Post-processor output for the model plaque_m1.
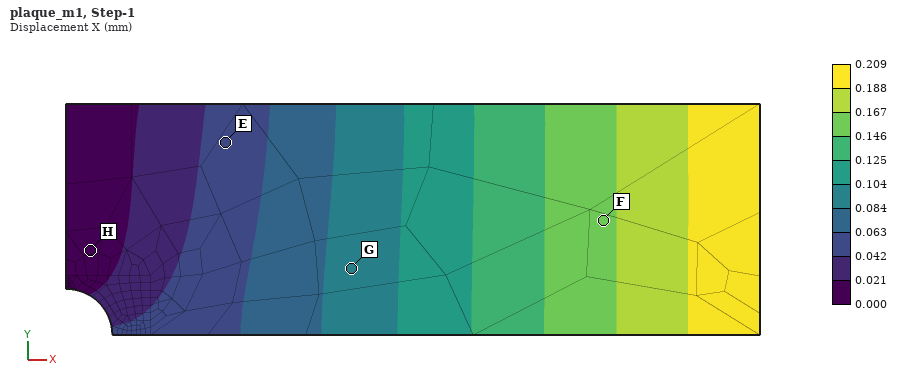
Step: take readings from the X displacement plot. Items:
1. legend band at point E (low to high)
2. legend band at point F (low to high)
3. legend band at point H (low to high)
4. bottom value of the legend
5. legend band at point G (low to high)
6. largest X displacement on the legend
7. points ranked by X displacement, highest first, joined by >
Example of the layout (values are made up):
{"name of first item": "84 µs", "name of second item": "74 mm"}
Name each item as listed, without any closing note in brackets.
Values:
{"legend band at point E": "0.042 to 0.063 mm", "legend band at point F": "0.146 to 0.167 mm", "legend band at point H": "0.000 to 0.021 mm", "bottom value of the legend": "0.000 mm", "legend band at point G": "0.084 to 0.104 mm", "largest X displacement on the legend": "0.209 mm", "points ranked by X displacement, highest first, joined by >": "F > G > E > H"}
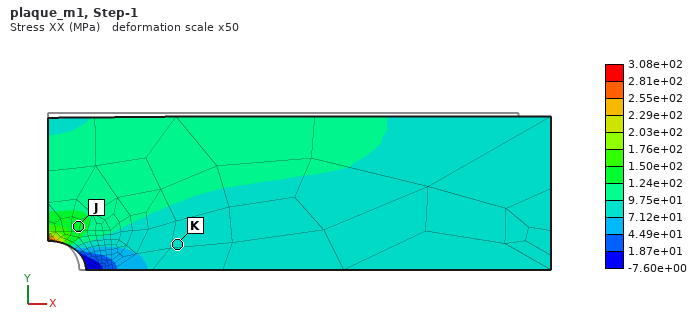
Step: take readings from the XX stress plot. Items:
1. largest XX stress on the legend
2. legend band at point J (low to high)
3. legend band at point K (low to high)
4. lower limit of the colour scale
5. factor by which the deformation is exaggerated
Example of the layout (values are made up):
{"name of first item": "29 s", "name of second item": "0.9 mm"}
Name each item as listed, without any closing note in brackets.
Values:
{"largest XX stress on the legend": "3.08e+02 MPa", "legend band at point J": "1.24e+02 to 1.50e+02 MPa", "legend band at point K": "7.12e+01 to 9.75e+01 MPa", "lower limit of the colour scale": "-7.60e+00 MPa", "factor by which the deformation is exaggerated": "50"}
